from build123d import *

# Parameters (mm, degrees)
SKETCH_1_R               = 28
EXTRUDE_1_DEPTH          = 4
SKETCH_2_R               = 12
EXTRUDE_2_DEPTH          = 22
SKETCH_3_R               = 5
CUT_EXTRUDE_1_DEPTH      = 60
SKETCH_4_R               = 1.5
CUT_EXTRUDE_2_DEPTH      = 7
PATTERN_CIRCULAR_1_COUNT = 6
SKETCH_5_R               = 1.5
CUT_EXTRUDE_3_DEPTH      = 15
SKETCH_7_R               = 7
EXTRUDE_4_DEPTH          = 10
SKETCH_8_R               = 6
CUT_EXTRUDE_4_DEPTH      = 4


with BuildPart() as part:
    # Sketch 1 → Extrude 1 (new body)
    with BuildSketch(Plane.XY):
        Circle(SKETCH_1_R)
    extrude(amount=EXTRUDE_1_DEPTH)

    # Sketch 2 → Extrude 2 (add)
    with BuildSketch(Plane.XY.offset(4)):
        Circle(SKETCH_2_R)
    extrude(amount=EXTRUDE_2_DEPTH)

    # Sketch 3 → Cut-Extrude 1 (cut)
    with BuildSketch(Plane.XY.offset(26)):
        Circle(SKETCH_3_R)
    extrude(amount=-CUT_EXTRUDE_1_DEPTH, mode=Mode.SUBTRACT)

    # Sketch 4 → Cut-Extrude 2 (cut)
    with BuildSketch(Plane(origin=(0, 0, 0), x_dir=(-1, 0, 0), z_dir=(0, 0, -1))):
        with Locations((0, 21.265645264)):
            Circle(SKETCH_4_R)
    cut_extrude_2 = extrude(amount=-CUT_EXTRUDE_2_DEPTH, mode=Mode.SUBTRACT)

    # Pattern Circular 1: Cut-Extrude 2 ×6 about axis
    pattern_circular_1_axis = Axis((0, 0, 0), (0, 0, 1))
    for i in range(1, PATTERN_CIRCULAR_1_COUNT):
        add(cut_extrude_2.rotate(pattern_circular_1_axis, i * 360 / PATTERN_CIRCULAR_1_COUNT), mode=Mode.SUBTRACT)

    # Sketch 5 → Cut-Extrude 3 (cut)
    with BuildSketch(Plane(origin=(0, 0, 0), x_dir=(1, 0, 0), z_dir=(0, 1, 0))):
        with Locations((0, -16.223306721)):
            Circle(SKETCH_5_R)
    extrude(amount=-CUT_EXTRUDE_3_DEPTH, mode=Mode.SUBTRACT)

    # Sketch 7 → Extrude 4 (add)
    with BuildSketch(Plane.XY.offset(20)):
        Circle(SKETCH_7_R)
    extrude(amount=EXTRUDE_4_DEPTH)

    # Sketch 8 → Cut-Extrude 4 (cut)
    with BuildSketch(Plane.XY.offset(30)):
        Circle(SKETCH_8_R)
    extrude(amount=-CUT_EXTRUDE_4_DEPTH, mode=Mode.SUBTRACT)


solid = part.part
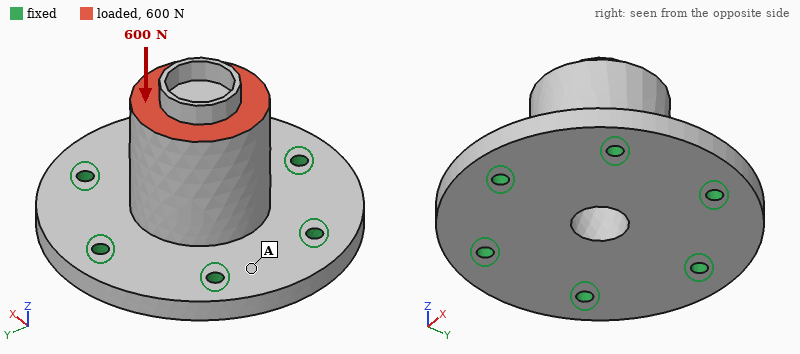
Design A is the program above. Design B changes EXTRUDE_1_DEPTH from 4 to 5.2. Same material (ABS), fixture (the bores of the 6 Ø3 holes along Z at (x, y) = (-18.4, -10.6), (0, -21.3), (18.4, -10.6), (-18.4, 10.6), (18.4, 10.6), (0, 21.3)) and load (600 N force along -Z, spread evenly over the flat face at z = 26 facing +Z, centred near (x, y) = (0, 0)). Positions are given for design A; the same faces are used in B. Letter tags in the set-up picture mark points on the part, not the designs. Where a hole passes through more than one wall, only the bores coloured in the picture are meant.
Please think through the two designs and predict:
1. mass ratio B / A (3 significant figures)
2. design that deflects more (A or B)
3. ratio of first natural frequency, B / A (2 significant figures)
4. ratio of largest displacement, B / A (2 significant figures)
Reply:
1.13
A
1.3
0.66
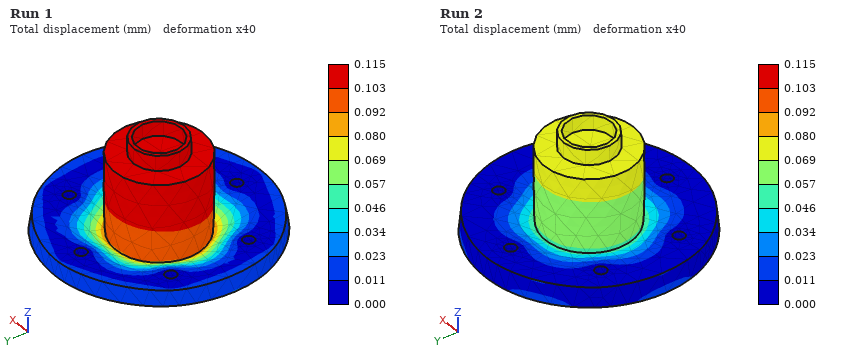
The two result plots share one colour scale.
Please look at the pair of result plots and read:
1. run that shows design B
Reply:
Run 2
